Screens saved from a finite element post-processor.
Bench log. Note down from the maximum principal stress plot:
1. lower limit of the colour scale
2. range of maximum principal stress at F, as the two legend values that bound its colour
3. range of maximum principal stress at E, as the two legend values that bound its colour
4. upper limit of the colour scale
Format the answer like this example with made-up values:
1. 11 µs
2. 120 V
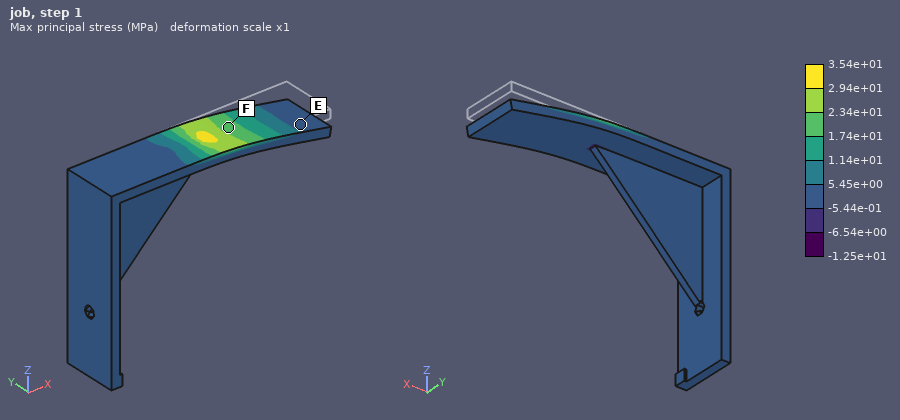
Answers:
1. -1.25e+01 MPa
2. 1.74e+01 to 2.34e+01 MPa
3. -5.44e-01 to 5.45e+00 MPa
4. 3.54e+01 MPa
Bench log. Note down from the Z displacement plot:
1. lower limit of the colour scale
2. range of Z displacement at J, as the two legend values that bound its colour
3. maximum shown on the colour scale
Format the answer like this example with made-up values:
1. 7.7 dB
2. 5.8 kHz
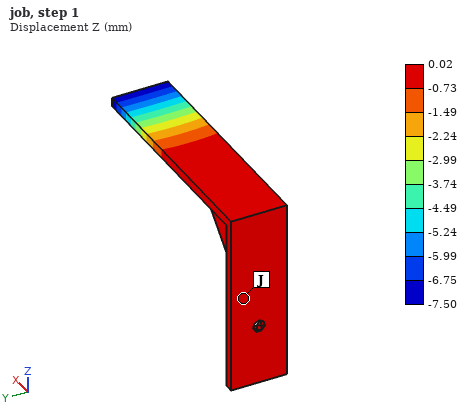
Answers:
1. -7.50 mm
2. -0.73 to 0.02 mm
3. 0.02 mm
